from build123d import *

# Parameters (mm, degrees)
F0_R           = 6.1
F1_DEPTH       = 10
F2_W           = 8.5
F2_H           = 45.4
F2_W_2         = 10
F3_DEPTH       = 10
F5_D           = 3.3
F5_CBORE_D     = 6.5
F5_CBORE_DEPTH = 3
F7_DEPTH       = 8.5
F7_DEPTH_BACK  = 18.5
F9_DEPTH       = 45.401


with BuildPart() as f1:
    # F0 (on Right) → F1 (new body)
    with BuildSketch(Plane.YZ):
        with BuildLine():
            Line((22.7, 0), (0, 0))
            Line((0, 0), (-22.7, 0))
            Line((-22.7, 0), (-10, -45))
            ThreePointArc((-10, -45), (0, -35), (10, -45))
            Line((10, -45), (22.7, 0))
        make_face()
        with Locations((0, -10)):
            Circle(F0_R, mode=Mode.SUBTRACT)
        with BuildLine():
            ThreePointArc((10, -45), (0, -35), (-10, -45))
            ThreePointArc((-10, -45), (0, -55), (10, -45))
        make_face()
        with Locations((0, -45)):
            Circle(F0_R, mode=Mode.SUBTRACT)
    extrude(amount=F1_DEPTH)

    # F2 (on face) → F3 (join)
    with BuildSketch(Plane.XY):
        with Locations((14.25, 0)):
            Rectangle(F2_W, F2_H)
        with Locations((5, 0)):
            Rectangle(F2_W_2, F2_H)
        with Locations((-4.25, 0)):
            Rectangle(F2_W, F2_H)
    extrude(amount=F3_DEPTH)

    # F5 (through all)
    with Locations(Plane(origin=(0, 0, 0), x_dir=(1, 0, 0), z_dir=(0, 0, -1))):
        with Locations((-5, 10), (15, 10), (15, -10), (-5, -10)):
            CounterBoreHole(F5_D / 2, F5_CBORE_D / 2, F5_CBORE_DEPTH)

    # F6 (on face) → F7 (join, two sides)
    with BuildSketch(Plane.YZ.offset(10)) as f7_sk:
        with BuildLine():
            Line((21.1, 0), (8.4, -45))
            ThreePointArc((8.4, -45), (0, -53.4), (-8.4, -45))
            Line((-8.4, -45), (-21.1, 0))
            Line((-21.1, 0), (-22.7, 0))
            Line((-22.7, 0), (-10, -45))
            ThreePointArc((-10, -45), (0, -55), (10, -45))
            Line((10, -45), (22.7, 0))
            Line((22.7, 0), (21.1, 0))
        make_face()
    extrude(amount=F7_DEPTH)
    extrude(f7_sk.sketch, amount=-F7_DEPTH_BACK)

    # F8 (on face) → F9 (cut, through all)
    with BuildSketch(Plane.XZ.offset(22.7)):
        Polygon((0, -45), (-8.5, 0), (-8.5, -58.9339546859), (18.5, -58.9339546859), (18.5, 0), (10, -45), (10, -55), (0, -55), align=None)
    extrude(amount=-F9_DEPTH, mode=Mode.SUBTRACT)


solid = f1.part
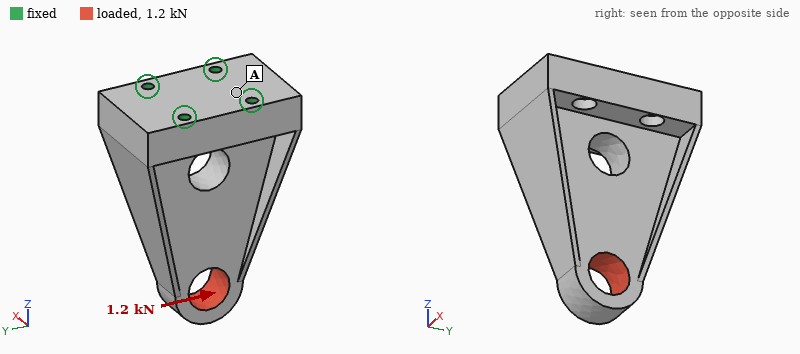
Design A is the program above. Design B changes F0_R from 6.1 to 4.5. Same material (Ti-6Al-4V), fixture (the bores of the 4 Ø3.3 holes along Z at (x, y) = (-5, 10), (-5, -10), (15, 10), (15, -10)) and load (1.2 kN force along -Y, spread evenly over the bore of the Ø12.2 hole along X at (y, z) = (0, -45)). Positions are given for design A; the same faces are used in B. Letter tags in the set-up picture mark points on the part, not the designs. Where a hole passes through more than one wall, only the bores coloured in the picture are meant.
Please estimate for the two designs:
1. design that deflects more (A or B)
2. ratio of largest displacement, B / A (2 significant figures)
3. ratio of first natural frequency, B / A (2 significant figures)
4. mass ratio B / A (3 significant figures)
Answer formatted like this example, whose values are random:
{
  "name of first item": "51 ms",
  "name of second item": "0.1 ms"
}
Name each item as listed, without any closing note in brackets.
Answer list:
{
  "design that deflects more": "A",
  "ratio of largest displacement, B / A": "0.88",
  "ratio of first natural frequency, B / A": "0.97",
  "mass ratio B / A": "1.04"
}
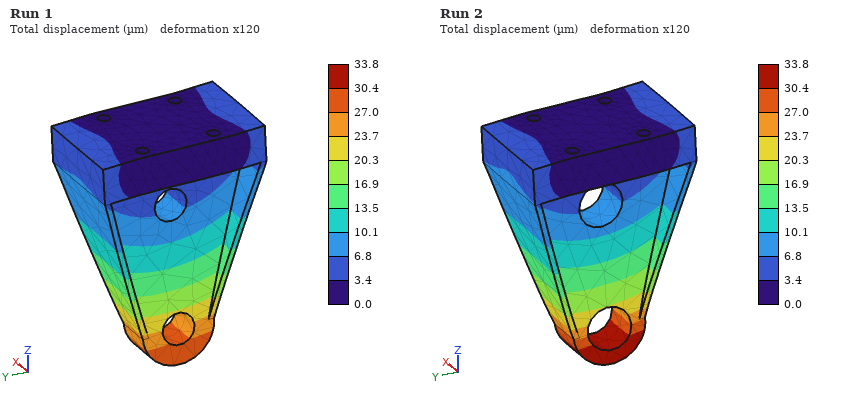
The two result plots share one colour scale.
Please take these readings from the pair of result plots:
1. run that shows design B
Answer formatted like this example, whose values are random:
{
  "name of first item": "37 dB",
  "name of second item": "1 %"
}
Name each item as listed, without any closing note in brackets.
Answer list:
{
  "run that shows design B": "Run 1"
}
